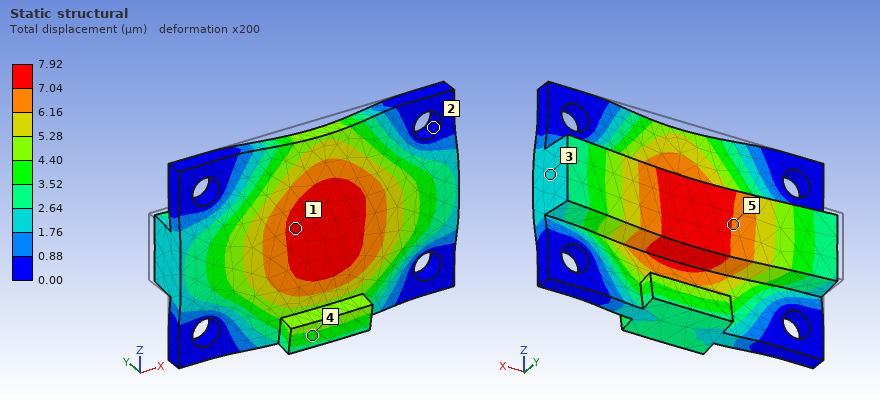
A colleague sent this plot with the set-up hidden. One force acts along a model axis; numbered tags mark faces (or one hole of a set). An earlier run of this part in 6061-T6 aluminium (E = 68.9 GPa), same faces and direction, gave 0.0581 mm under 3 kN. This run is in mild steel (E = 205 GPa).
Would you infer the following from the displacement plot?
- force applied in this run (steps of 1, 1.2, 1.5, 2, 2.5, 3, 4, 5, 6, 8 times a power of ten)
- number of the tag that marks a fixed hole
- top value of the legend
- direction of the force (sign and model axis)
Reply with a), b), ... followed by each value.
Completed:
a) 1.2 kN
b) 2
c) 7.92 µm
d) -Y
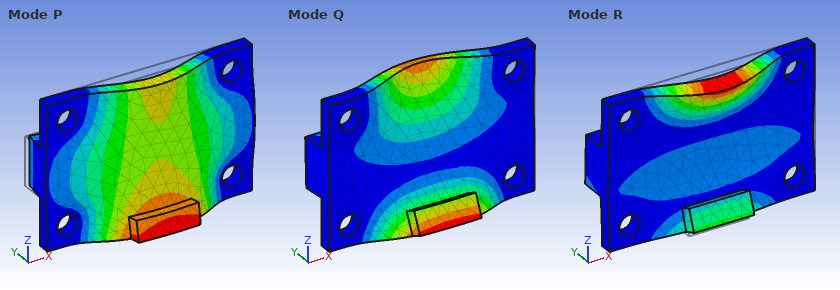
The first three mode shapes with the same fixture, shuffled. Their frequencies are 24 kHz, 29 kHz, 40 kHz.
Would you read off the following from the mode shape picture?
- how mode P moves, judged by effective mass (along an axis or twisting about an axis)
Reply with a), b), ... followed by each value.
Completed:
a) along Y
